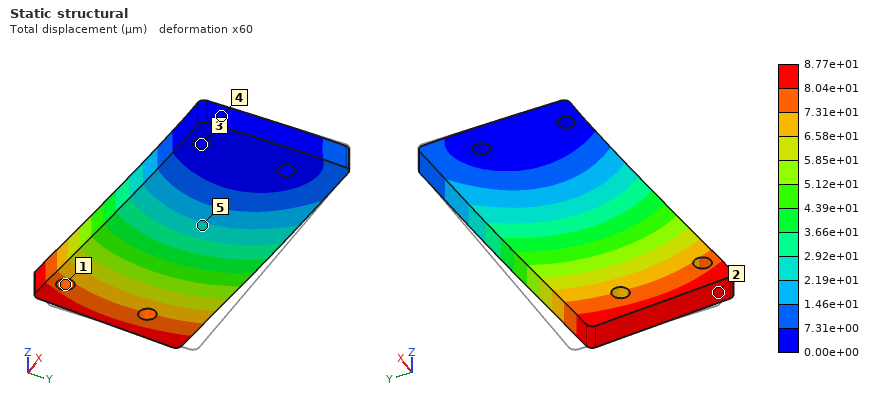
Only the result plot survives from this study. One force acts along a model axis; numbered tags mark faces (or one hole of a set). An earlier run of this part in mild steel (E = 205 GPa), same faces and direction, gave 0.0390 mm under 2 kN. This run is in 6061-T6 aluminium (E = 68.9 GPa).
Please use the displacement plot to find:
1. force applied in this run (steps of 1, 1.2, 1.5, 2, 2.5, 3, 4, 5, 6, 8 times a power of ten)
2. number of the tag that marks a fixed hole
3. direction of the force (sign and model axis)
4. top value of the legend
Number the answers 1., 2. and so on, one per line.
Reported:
1. 1.5 kN
2. 3
3. -Y
4. 8.77e+01 µm
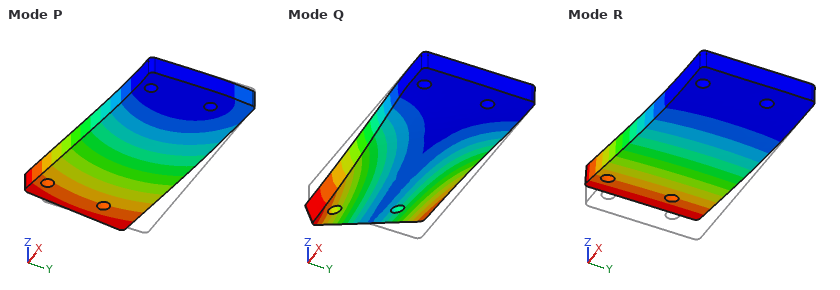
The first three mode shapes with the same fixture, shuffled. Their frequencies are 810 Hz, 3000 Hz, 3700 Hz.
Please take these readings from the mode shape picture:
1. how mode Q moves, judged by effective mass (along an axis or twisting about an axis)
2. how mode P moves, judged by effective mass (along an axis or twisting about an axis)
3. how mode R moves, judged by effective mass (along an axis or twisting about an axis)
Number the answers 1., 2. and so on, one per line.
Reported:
1. twisting about X
2. along Y
3. along Z
